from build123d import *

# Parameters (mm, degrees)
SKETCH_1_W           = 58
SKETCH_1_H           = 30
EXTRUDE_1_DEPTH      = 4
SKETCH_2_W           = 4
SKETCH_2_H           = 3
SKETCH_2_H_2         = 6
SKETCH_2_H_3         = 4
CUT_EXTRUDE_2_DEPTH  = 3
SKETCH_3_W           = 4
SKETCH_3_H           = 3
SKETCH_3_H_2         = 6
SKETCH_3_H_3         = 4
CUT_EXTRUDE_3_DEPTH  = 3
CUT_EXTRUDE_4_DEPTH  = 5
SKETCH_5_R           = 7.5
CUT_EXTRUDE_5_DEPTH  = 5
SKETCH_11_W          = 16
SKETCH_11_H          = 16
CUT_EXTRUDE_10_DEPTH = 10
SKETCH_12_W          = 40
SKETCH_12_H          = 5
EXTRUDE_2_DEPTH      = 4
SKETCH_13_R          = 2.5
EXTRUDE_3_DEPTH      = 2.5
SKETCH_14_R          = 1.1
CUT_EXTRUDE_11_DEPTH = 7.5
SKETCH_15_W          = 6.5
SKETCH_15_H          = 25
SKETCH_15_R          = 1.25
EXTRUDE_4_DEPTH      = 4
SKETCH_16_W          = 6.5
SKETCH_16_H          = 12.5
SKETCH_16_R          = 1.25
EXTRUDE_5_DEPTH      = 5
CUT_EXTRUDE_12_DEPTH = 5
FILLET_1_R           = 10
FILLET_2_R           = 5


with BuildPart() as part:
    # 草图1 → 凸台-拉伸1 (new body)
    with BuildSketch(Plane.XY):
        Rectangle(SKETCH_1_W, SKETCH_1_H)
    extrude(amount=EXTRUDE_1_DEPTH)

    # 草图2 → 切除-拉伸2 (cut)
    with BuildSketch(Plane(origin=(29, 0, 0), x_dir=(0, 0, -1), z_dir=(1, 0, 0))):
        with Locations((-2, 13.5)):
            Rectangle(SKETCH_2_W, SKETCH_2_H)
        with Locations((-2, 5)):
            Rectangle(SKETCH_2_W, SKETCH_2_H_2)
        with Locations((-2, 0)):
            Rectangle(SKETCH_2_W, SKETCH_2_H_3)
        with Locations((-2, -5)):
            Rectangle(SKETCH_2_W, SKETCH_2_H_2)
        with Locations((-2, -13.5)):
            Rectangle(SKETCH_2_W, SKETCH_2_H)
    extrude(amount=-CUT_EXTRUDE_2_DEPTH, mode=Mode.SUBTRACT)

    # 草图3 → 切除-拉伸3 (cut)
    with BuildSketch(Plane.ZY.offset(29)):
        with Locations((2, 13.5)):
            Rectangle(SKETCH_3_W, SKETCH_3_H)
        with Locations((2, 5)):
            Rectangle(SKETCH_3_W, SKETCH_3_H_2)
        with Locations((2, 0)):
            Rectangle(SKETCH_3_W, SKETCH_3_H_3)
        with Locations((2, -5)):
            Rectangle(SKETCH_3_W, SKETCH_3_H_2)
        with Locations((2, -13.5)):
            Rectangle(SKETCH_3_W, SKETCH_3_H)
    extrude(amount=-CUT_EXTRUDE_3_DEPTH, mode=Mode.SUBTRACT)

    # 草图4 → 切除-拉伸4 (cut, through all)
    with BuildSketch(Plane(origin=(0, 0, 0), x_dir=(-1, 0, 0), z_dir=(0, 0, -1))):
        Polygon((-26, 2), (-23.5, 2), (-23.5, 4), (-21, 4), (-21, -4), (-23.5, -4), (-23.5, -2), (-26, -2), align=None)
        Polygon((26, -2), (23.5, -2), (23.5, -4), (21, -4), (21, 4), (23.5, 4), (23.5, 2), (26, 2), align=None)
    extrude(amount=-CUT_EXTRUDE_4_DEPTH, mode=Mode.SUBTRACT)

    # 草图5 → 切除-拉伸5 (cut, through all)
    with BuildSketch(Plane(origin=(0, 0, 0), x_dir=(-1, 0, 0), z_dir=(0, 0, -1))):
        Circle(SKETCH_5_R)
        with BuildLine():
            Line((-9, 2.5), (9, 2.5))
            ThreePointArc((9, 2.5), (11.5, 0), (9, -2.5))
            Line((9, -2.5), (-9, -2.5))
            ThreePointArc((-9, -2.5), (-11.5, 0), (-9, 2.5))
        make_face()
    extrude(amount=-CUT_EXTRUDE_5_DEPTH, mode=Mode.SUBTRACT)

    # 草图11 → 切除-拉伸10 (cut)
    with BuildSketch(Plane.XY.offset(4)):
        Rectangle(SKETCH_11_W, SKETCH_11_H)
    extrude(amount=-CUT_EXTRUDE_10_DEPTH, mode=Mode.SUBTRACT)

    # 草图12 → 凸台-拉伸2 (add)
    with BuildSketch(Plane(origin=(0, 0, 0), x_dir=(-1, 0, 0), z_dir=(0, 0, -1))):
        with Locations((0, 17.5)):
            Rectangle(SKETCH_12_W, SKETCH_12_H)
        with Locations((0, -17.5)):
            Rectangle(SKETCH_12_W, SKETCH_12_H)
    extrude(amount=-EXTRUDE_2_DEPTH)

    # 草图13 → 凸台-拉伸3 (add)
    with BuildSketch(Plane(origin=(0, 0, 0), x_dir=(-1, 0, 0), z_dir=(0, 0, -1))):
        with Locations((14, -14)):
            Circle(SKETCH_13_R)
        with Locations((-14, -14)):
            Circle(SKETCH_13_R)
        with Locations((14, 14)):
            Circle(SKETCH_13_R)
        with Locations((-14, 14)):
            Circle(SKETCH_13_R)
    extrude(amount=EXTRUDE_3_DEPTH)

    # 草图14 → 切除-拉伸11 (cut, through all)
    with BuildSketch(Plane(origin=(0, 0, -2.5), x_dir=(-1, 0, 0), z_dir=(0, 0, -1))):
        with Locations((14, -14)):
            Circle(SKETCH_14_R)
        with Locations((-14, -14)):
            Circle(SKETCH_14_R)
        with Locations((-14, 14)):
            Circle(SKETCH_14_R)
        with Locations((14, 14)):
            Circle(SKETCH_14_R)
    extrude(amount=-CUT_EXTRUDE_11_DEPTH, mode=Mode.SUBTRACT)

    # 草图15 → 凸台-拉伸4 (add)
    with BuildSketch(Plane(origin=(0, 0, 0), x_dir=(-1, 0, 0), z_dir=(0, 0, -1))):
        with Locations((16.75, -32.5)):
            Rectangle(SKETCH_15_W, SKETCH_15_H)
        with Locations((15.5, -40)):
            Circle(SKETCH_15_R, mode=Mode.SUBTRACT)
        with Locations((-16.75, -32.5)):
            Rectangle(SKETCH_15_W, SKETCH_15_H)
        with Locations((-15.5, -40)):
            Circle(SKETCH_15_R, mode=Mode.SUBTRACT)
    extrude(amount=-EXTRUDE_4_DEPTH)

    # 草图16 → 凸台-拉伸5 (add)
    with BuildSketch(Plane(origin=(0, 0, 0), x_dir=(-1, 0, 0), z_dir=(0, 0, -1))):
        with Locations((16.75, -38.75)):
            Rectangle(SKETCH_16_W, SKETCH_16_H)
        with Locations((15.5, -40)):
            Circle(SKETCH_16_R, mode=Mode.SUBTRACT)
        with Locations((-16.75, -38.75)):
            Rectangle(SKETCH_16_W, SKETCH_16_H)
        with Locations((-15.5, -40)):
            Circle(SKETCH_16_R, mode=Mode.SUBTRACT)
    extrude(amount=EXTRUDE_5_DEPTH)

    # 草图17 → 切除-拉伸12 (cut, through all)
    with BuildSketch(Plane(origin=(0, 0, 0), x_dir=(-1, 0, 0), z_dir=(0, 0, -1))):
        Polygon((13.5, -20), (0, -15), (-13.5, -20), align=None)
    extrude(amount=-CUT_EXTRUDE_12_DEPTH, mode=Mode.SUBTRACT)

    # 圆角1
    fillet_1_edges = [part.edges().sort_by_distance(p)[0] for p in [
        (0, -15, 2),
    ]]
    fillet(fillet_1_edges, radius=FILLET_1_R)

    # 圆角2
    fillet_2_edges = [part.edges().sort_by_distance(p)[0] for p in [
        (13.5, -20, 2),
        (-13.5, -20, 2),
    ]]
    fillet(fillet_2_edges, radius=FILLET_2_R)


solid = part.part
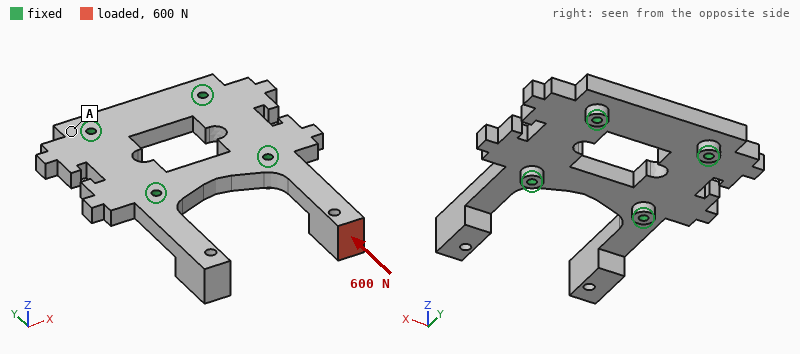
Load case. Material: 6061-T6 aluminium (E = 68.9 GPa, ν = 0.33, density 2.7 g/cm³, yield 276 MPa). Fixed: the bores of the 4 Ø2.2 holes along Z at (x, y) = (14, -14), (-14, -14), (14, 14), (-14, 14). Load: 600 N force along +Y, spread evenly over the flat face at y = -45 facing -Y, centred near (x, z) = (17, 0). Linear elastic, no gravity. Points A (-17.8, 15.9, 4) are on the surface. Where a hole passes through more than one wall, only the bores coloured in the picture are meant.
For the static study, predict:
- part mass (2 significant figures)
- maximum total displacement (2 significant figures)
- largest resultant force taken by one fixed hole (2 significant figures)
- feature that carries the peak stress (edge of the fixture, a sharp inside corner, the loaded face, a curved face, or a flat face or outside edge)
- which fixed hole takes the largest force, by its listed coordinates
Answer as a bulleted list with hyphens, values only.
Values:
- 23 g
- 0.24 mm
- 540 N
- a curved face
- (14, -14)
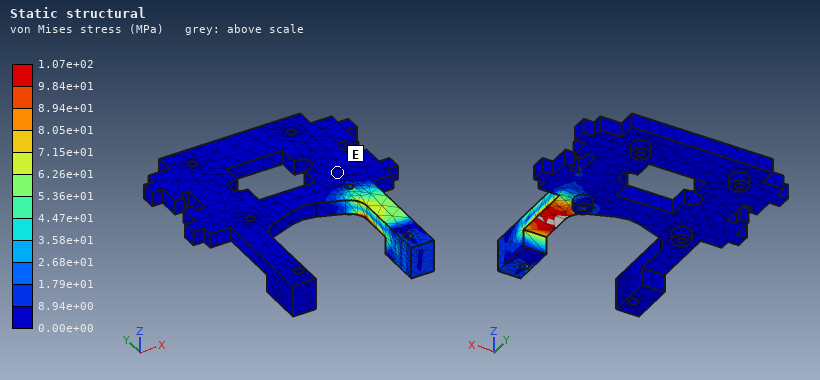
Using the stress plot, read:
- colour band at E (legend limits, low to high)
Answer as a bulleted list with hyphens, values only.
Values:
- 0.00e+00 to 8.94e+00 MPa
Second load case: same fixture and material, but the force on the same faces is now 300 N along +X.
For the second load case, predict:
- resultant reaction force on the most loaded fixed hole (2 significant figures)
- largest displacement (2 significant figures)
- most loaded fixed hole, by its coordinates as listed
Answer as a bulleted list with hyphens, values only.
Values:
- 480 N
- 0.39 mm
- (14, -14)
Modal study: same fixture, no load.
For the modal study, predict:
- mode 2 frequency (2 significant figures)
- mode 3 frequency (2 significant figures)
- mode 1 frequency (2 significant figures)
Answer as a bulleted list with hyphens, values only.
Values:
- 2600 Hz
- 4400 Hz
- 2600 Hz
